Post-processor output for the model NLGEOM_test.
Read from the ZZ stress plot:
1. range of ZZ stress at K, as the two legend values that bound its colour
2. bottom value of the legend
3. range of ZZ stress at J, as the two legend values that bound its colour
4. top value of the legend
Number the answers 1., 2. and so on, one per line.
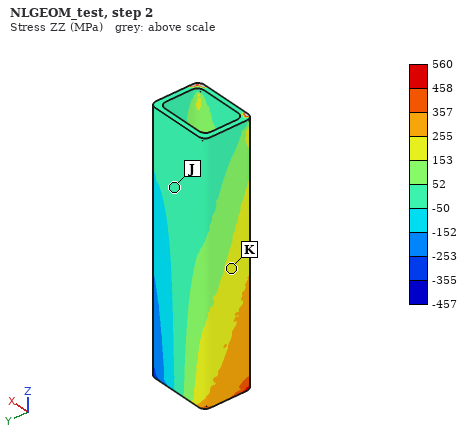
1. 153 to 255 MPa
2. -457 MPa
3. -50 to 52 MPa
4. 560 MPa
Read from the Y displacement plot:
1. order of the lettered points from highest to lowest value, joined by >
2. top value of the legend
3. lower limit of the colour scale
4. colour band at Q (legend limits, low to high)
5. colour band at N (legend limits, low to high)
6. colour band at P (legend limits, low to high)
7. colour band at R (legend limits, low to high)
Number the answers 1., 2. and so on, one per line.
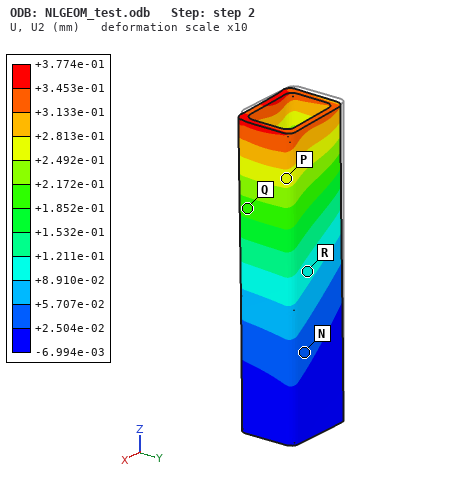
1. P > Q > R > N
2. +3.774e-01 mm
3. -6.994e-03 mm
4. +1.852e-01 to +2.172e-01 mm
5. +2.504e-02 to +5.707e-02 mm
6. +2.492e-01 to +2.813e-01 mm
7. +8.910e-02 to +1.211e-01 mm
